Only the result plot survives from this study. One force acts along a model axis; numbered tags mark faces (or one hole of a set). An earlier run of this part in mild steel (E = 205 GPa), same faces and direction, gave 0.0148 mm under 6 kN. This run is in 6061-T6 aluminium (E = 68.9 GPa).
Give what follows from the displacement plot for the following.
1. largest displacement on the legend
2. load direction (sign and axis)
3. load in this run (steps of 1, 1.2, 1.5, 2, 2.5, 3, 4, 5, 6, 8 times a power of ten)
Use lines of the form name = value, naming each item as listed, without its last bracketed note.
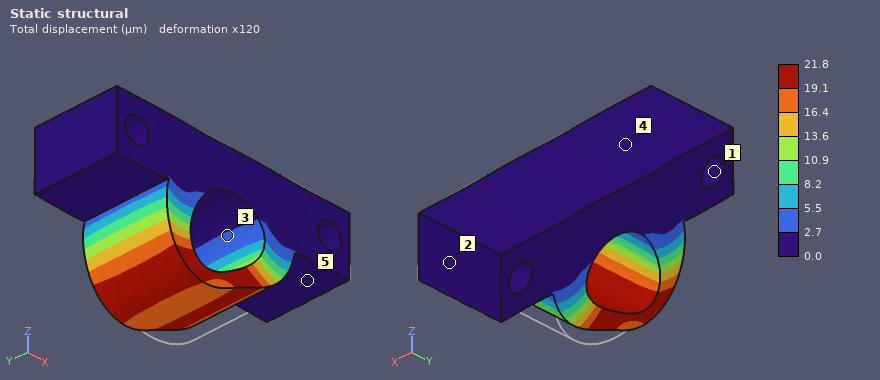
largest displacement on the legend = 21.8 µm
load direction = -X
load in this run = 3 kN
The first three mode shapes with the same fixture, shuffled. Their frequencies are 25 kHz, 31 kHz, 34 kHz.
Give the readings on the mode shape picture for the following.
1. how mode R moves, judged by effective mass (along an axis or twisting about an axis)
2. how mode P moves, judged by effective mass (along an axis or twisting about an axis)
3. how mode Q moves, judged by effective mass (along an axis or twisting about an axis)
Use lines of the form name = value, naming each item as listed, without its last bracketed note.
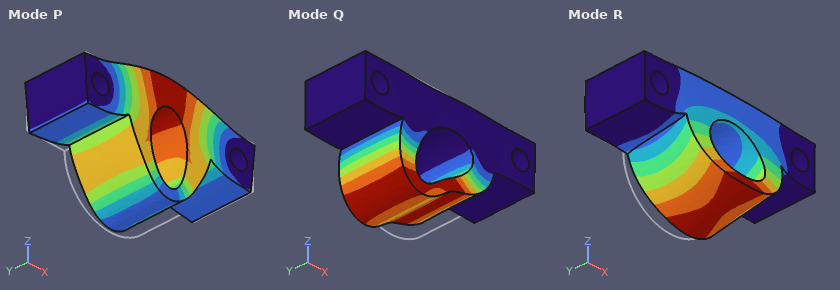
how mode R moves, judged by effective mass = along Y
how mode P moves, judged by effective mass = along Z
how mode Q moves, judged by effective mass = along X
